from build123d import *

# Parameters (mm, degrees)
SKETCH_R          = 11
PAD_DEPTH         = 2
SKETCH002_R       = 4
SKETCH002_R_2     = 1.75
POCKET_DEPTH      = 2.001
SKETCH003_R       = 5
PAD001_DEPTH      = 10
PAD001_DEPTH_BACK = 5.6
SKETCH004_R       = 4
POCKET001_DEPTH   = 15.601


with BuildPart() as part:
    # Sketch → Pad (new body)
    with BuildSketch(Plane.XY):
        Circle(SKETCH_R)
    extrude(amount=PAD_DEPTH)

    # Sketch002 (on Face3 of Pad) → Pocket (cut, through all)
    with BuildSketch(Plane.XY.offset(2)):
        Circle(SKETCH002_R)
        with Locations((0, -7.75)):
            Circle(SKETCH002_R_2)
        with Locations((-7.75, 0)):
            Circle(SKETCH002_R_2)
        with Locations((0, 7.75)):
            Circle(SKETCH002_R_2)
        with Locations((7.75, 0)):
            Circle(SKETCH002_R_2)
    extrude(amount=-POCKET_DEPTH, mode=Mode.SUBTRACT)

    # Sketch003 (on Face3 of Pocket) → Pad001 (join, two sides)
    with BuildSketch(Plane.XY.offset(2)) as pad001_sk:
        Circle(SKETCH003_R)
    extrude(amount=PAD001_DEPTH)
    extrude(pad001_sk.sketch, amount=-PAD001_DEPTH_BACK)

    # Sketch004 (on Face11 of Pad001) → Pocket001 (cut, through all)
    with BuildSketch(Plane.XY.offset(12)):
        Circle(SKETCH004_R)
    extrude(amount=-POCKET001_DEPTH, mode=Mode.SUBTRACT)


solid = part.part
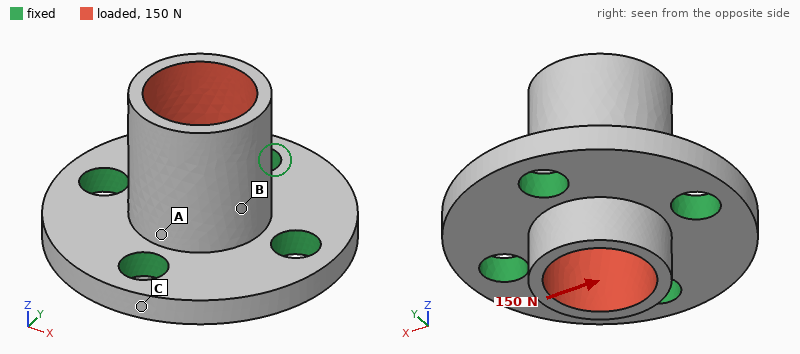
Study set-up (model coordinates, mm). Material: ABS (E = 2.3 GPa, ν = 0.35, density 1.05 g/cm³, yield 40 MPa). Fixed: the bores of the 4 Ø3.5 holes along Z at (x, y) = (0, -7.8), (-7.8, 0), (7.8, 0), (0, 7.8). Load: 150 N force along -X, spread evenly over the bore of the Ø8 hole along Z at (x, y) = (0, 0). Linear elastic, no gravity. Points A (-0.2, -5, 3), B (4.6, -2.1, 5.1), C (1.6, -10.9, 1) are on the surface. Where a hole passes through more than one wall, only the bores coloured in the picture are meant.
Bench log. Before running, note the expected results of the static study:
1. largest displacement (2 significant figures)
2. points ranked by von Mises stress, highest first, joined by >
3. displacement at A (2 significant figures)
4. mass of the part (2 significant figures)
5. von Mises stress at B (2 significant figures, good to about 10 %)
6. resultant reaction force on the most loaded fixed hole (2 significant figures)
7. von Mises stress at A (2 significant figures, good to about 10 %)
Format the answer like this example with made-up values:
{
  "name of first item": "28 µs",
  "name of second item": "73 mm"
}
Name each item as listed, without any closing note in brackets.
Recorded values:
{
  "largest displacement": "93 µm",
  "points ranked by von Mises stress, highest first, joined by >": "A > B > C",
  "displacement at A": "16 µm",
  "mass of the part": "1.0 g",
  "von Mises stress at B": "3.7 MPa",
  "resultant reaction force on the most loaded fixed hole": "56 N",
  "von Mises stress at A": "6.2 MPa"
}
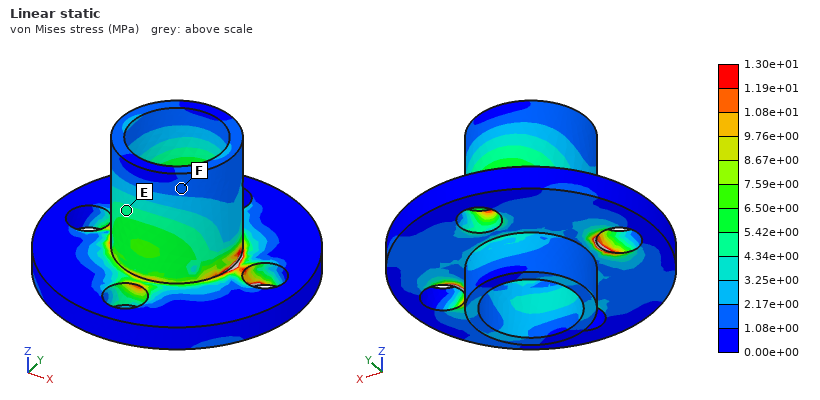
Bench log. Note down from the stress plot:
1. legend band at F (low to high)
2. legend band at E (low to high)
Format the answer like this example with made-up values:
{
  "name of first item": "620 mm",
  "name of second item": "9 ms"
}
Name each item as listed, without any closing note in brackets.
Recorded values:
{
  "legend band at F": "1.08e+00 to 2.17e+00 MPa",
  "legend band at E": "4.34e+00 to 5.42e+00 MPa"
}
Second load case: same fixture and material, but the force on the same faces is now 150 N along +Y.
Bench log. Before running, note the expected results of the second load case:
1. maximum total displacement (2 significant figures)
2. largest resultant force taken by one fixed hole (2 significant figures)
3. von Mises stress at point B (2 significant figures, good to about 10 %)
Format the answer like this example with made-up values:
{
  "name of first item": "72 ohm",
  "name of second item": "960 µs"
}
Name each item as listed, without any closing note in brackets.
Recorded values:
{
  "maximum total displacement": "93 µm",
  "largest resultant force taken by one fixed hole": "56 N",
  "von Mises stress at point B": "6.3 MPa"
}
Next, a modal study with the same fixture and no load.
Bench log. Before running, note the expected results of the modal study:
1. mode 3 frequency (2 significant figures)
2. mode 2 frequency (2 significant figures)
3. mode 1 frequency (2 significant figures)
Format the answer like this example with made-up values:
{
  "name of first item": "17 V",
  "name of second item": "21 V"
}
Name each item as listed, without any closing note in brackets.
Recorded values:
{
  "mode 3 frequency": "11 kHz",
  "mode 2 frequency": "11 kHz",
  "mode 1 frequency": "11 kHz"
}
